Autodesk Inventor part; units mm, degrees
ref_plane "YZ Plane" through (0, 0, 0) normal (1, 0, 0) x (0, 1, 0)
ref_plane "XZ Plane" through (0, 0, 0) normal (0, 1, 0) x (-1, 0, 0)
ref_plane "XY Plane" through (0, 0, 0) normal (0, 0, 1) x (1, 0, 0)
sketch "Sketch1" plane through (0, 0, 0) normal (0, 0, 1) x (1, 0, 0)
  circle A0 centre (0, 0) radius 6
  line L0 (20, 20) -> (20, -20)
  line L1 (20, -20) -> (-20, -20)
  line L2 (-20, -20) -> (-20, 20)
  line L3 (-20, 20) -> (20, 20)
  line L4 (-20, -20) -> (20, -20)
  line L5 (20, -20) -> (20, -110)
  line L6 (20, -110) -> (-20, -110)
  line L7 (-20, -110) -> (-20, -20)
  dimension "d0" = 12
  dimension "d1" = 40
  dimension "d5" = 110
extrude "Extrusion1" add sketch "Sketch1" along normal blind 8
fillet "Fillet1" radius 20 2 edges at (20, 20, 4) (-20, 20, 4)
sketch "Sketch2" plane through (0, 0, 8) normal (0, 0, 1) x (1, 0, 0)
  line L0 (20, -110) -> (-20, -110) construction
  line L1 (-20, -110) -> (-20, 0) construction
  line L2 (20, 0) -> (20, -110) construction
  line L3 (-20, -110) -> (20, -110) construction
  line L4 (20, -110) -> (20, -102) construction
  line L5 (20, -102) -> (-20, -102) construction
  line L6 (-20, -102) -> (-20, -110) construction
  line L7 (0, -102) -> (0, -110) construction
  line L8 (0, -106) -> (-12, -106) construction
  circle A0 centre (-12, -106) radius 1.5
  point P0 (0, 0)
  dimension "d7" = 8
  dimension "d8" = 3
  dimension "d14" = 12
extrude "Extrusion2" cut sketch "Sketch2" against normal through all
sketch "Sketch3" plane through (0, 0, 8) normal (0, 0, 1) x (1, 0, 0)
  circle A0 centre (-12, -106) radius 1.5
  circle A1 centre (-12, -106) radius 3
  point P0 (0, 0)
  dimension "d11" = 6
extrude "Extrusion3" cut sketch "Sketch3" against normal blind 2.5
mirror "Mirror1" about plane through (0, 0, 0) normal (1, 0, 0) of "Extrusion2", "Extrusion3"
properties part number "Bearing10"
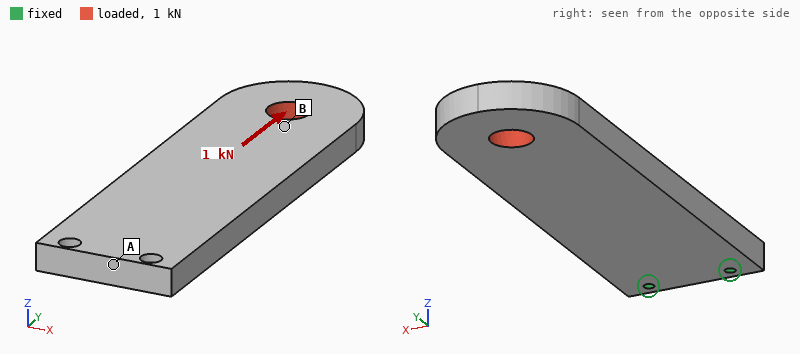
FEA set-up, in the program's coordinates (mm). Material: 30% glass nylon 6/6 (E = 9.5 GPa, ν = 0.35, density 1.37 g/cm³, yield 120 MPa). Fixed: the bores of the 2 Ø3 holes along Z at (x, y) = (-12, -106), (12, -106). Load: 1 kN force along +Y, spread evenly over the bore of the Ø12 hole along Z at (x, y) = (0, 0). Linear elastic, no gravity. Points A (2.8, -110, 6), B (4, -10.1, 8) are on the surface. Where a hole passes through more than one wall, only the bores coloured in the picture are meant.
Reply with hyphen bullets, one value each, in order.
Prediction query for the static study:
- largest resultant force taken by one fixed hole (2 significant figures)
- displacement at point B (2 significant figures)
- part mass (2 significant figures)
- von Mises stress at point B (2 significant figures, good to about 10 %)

- 500 N
- 0.11 mm
- 54 g
- 4.2 MPa
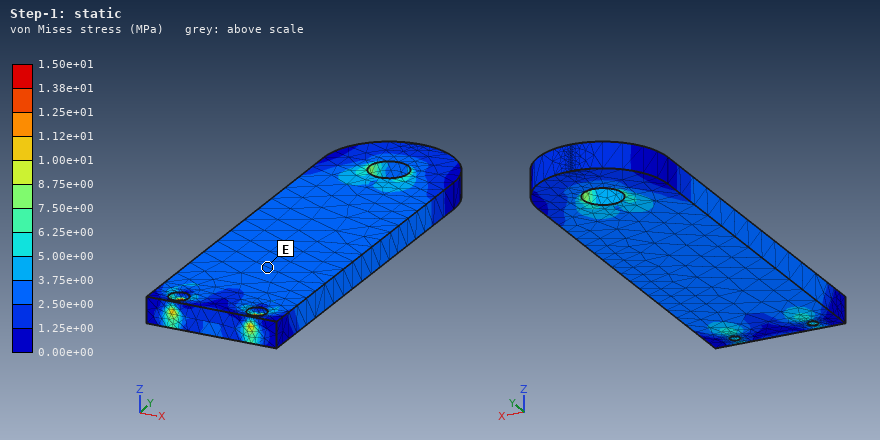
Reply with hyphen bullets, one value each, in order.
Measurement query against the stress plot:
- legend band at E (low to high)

- 2.50e+00 to 3.75e+00 MPa
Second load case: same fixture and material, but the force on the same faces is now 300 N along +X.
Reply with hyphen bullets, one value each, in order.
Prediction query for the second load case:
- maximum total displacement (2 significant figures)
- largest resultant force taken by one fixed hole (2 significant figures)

- 0.53 mm
- 1.3 kN
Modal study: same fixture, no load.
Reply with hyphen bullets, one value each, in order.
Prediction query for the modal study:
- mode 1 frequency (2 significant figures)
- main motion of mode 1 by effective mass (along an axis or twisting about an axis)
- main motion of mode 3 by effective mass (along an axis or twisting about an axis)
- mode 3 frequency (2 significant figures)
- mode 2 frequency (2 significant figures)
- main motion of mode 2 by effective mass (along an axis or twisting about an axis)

- 200 Hz
- along Z
- along Z
- 1300 Hz
- 940 Hz
- along X
